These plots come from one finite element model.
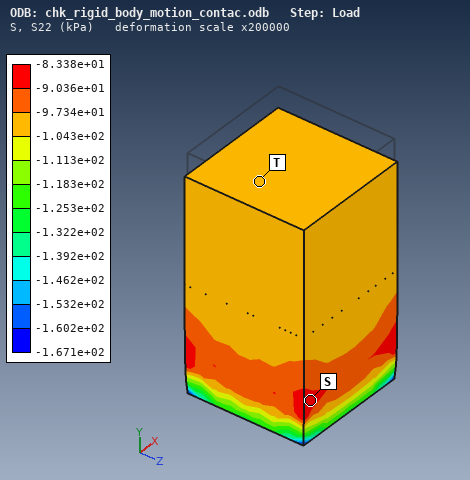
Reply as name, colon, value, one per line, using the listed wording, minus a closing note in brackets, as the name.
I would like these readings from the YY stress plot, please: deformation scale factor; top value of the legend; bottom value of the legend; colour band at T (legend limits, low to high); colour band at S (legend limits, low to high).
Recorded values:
deformation scale factor: 200000
top value of the legend: -8.338e+01 kPa
bottom value of the legend: -1.671e+02 kPa
colour band at T: -1.043e+02 to -9.734e+01 kPa
colour band at S: -9.036e+01 to -8.338e+01 kPa
